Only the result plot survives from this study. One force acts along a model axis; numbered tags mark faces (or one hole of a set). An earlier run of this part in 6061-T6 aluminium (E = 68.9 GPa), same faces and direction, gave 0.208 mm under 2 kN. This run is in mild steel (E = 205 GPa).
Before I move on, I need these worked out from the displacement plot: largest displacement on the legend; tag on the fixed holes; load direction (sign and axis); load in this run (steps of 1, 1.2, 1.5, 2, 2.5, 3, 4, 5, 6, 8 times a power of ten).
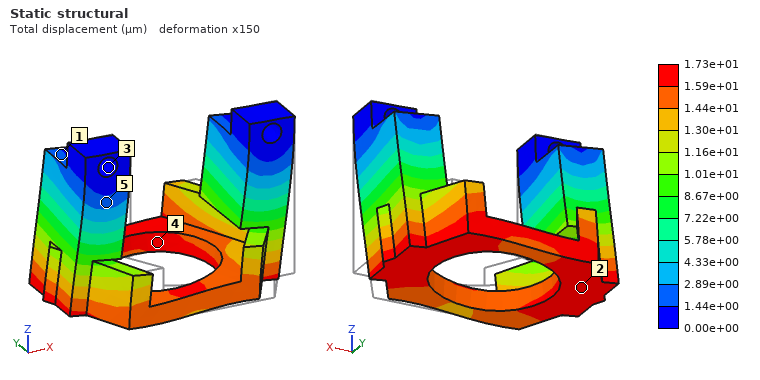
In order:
1.73e+01 µm
3
-X
500 N
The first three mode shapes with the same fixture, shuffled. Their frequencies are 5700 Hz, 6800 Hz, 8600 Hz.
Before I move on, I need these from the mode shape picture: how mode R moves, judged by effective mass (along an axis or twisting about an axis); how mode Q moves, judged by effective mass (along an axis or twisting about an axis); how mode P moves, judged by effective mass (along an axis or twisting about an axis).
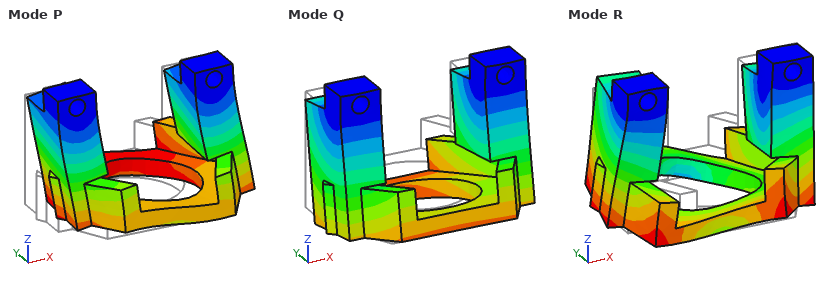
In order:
twisting about Z
along Y
along X
